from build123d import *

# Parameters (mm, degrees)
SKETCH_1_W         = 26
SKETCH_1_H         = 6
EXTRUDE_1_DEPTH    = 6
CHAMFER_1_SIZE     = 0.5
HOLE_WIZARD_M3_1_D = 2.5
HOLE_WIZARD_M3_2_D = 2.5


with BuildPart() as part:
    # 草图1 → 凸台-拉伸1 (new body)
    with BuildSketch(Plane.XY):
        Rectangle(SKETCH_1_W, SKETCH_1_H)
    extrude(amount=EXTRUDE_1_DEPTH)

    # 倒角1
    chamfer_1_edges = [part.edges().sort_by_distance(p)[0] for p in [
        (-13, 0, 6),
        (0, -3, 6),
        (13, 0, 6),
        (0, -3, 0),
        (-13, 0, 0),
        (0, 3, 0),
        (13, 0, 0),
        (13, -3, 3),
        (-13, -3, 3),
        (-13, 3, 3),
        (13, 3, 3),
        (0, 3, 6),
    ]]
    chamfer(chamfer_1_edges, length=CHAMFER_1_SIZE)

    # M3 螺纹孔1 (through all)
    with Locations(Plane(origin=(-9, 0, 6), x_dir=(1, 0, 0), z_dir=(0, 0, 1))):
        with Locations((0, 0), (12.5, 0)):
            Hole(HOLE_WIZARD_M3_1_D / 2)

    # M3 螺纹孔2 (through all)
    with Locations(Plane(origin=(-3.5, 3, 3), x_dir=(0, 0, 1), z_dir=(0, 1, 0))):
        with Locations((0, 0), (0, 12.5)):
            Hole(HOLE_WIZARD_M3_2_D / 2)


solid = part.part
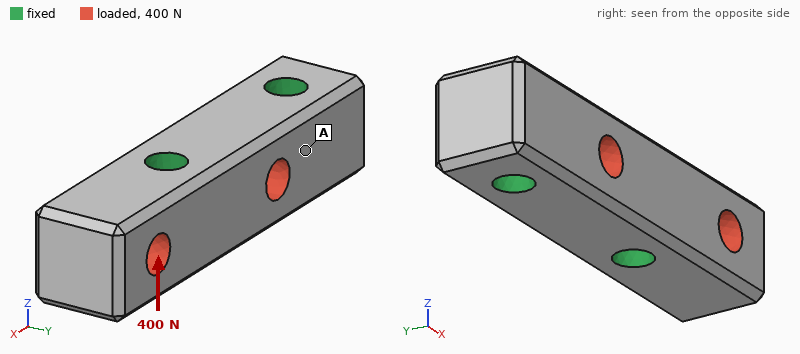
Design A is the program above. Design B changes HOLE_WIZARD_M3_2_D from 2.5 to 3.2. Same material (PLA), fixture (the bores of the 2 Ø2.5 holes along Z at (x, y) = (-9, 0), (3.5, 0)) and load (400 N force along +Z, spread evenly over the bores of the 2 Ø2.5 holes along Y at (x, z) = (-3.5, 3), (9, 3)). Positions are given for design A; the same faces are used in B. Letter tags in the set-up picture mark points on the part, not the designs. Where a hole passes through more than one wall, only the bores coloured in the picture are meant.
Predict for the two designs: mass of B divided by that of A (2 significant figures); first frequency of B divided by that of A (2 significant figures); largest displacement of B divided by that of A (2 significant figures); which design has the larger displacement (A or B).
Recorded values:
0.95
0.98
1.2
B
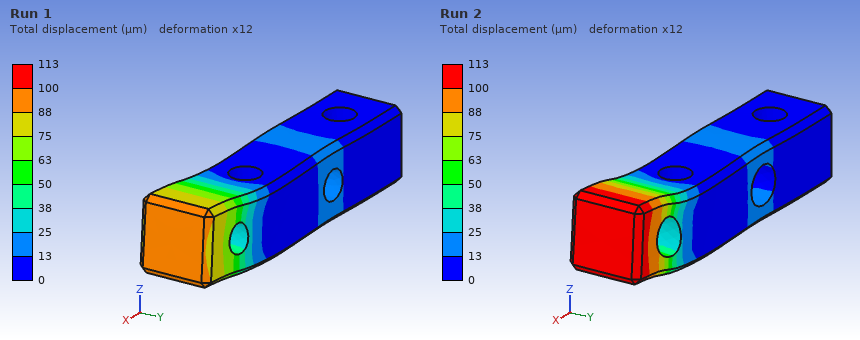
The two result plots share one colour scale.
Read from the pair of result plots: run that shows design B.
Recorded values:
Run 2
